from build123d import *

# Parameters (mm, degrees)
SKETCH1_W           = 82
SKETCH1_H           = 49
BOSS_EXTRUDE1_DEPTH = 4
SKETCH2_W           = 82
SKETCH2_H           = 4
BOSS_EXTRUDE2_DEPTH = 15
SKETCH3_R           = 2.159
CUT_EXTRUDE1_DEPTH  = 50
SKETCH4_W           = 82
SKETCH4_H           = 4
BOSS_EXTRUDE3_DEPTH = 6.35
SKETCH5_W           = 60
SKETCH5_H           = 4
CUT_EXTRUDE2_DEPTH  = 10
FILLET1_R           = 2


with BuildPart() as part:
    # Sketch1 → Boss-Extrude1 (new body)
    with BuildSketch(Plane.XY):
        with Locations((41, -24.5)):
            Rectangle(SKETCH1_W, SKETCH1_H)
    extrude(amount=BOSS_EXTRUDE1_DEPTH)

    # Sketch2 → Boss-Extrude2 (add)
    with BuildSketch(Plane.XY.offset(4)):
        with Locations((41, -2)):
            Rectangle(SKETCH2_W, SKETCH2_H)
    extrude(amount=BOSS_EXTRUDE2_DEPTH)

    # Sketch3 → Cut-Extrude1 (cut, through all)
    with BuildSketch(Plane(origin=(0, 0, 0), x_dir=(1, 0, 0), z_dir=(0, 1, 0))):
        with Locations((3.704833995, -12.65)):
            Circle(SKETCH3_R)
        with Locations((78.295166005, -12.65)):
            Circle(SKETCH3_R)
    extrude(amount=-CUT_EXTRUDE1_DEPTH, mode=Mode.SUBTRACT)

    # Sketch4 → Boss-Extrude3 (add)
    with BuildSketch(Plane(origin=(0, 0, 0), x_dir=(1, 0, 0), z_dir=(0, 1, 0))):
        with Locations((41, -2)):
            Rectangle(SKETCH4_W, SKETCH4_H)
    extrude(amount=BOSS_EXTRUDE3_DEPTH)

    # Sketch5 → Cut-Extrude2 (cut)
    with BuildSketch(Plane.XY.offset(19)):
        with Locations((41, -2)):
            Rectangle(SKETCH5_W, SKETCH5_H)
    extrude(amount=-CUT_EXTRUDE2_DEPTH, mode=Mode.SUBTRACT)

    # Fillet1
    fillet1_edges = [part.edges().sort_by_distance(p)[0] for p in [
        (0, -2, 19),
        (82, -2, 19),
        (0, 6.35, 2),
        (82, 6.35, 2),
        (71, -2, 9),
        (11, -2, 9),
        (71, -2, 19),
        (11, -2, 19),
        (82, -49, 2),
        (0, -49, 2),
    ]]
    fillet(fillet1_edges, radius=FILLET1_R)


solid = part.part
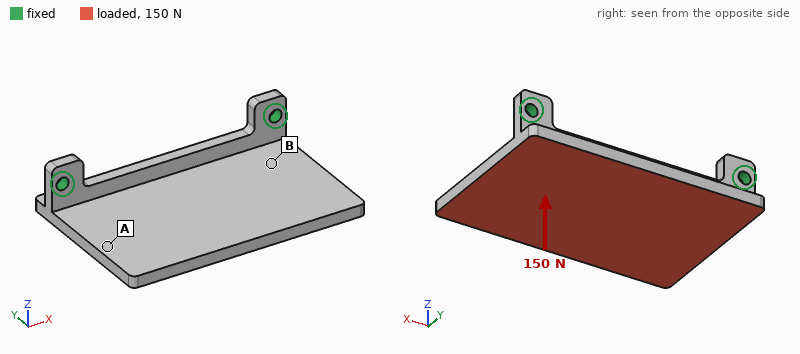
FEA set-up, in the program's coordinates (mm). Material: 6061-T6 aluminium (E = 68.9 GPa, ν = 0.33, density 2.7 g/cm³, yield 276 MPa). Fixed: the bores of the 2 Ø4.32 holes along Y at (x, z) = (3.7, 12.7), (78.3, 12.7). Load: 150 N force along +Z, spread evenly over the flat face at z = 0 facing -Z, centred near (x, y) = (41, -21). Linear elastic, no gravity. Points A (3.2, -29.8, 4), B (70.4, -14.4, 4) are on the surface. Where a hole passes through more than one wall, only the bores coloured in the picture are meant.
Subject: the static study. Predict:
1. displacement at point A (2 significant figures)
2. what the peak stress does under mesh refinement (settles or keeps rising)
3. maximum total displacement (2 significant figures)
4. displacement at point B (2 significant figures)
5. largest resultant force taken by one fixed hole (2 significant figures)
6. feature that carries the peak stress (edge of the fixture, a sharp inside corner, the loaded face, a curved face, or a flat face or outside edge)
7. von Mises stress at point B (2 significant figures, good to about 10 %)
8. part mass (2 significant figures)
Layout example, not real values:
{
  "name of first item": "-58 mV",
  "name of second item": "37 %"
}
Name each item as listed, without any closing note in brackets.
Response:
{
  "displacement at point A": "0.10 mm",
  "what the peak stress does under mesh refinement": "keeps rising",
  "maximum total displacement": "0.20 mm",
  "displacement at point B": "0.043 mm",
  "largest resultant force taken by one fixed hole": "100 N",
  "feature that carries the peak stress": "edge of the fixture",
  "von Mises stress at point B": "8.3 MPa",
  "part mass": "55 g"
}
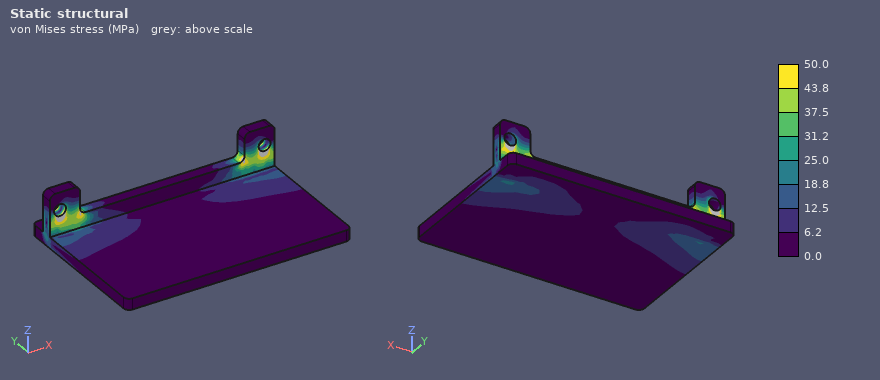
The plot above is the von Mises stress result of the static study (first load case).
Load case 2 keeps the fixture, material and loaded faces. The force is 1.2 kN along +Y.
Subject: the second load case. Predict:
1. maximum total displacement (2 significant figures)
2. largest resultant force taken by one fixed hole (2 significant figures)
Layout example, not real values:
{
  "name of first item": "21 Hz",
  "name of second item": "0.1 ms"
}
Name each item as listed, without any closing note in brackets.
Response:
{
  "maximum total displacement": "0.47 mm",
  "largest resultant force taken by one fixed hole": "600 N"
}
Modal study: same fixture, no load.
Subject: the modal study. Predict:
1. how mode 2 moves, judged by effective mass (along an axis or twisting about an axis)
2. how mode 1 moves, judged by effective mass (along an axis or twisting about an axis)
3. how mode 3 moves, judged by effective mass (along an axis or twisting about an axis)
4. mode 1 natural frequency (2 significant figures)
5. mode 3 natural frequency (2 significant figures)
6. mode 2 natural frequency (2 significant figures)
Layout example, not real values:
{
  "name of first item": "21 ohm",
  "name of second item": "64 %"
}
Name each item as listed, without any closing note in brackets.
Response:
{
  "how mode 2 moves, judged by effective mass": "twisting about Y",
  "how mode 1 moves, judged by effective mass": "along Z",
  "how mode 3 moves, judged by effective mass": "along Y",
  "mode 1 natural frequency": "750 Hz",
  "mode 3 natural frequency": "4300 Hz",
  "mode 2 natural frequency": "2100 Hz"
}
